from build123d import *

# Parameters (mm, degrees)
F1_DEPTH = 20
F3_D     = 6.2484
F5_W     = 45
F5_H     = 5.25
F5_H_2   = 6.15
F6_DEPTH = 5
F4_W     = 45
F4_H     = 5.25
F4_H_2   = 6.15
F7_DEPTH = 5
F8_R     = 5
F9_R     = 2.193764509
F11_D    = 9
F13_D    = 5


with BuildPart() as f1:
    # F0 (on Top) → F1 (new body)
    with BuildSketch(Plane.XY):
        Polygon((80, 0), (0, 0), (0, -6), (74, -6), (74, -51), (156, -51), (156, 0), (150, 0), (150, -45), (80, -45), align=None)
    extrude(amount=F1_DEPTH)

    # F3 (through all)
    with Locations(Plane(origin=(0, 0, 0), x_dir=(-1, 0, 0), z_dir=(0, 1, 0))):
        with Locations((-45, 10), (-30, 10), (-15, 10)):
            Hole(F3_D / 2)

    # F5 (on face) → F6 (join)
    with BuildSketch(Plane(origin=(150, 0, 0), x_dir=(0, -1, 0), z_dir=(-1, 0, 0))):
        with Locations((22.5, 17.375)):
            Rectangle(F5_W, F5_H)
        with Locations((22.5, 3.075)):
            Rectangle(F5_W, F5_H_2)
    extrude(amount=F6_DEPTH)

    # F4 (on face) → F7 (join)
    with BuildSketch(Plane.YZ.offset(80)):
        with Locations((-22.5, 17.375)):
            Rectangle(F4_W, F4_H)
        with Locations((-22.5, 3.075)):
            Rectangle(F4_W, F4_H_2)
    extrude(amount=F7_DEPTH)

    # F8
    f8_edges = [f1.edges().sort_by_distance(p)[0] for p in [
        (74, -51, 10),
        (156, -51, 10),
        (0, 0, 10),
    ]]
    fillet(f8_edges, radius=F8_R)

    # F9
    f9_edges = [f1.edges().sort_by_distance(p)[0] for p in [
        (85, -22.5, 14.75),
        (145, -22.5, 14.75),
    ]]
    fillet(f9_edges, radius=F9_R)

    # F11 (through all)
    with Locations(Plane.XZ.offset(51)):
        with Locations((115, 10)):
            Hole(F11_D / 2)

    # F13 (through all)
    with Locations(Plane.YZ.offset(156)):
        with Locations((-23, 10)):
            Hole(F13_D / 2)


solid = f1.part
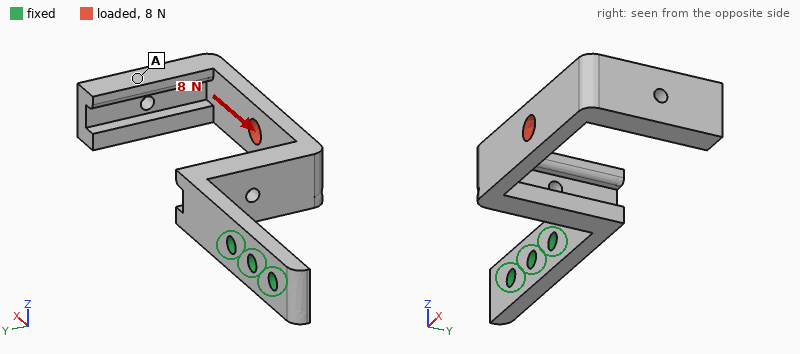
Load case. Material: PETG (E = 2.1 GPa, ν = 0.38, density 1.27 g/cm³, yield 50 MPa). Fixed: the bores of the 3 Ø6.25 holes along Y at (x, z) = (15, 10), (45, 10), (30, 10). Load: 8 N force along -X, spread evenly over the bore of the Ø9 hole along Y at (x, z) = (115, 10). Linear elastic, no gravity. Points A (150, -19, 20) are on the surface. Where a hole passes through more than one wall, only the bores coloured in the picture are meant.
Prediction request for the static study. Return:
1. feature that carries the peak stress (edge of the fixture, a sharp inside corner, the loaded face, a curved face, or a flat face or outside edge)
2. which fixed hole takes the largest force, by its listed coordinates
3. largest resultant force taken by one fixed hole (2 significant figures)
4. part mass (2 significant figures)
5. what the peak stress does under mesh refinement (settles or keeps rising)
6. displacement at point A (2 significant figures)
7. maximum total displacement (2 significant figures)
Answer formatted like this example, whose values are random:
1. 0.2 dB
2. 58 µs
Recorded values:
1. edge of the fixture
2. (45, 10)
3. 8.0 N
4. 42 g
5. keeps rising
6. 1.4 mm
7. 1.7 mm
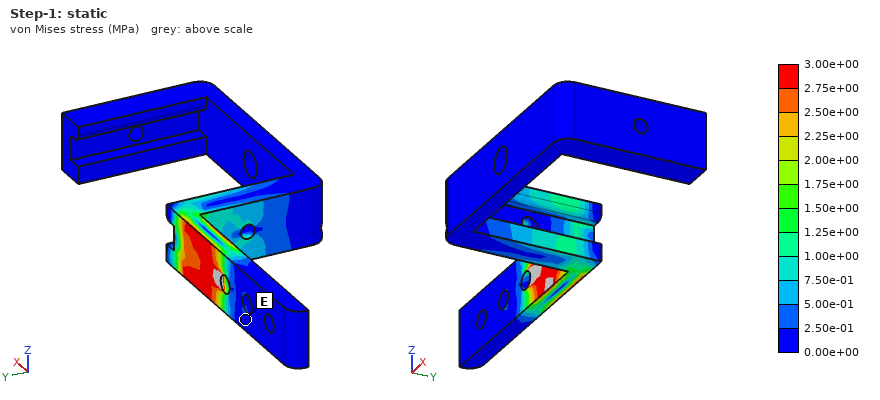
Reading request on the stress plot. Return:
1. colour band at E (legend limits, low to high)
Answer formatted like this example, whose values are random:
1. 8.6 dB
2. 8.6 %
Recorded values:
1. 0.00e+00 to 2.50e-01 MPa
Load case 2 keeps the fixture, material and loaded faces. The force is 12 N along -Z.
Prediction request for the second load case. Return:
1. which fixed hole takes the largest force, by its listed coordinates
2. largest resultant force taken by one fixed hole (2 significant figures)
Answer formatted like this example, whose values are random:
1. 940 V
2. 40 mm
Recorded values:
1. (45, 10)
2. 36 N
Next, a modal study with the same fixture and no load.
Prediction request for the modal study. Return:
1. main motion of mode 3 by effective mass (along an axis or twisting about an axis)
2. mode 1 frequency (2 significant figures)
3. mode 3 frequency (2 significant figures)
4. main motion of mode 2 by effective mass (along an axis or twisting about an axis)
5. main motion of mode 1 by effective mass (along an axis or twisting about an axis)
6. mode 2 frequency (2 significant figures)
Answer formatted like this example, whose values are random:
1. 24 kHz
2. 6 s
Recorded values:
1. along X
2. 53 Hz
3. 140 Hz
4. along Z
5. along Y
6. 84 Hz
